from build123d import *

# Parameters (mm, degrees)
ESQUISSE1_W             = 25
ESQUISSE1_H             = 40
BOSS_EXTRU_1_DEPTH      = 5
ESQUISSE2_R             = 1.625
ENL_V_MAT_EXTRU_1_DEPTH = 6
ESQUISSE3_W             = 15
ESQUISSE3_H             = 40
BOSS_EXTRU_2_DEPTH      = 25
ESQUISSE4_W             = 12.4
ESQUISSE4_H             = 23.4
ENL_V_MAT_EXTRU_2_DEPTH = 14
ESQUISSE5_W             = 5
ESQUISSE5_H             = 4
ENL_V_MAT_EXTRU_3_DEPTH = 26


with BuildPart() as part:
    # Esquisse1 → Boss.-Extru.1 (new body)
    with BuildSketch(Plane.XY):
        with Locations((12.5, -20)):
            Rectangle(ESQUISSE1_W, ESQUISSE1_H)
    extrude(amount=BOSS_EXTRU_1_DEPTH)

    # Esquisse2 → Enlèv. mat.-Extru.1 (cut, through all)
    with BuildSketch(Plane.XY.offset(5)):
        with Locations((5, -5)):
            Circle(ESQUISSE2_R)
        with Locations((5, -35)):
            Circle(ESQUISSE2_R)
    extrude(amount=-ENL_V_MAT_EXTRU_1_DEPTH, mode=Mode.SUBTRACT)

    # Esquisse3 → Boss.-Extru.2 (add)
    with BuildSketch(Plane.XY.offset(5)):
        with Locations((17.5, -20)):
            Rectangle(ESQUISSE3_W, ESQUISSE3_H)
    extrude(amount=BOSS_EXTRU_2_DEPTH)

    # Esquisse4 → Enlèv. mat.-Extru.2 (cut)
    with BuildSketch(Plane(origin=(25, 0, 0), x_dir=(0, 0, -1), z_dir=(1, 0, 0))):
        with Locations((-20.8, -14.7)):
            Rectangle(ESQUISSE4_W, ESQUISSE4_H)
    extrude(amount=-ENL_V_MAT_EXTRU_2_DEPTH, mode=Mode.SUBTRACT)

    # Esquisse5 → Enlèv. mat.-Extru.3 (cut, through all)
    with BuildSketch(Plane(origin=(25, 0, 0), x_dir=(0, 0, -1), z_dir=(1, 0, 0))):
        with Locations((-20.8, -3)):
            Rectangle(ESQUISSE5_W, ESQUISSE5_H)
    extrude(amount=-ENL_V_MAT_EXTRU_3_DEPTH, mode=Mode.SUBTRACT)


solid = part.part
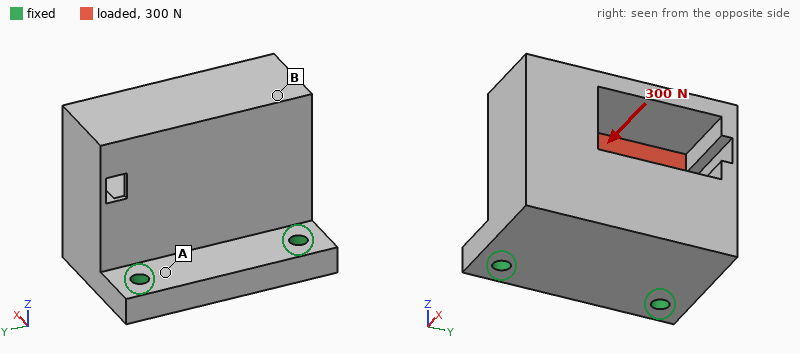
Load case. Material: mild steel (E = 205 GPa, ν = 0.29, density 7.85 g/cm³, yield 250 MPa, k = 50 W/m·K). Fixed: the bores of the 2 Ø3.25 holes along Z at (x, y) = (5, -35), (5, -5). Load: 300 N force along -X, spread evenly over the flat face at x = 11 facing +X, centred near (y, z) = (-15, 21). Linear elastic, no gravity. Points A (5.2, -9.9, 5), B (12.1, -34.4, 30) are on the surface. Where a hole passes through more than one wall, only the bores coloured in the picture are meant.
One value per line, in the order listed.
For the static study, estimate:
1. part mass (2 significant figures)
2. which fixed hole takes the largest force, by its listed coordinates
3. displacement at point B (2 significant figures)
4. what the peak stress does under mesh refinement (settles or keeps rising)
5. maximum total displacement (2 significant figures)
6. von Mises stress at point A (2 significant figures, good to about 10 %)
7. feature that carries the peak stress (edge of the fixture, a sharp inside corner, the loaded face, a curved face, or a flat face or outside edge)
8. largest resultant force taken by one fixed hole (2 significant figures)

120 g
(5, -5)
18 µm
keeps rising
22 µm
23 MPa
edge of the fixture
200 N
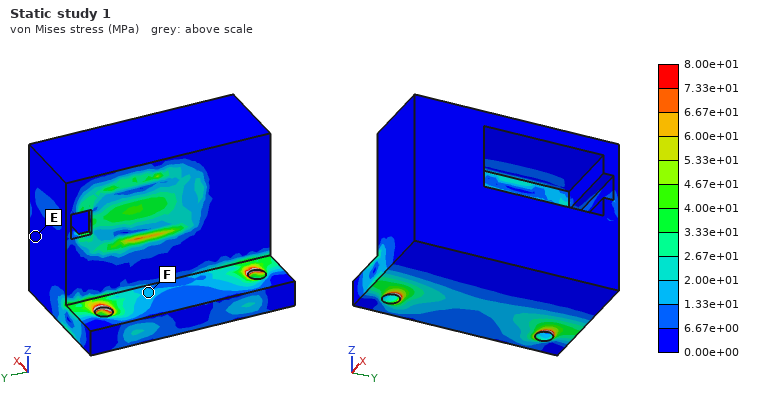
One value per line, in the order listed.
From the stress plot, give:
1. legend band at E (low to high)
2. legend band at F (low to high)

0.00e+00 to 6.67e+00 MPa
1.33e+01 to 2.00e+01 MPa
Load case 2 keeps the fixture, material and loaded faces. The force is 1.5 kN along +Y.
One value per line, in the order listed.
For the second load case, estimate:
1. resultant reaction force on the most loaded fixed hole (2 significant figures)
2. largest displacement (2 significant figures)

1.2 kN
12 µm
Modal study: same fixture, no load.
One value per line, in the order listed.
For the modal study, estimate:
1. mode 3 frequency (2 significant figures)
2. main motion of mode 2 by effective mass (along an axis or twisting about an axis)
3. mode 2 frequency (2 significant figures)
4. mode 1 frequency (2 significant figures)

12 kHz
along Y
8200 Hz
2600 Hz
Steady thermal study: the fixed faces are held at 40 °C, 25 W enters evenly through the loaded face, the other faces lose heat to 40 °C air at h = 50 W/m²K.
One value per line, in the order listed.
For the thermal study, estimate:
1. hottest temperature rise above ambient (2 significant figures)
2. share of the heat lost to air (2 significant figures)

82 K
34 %
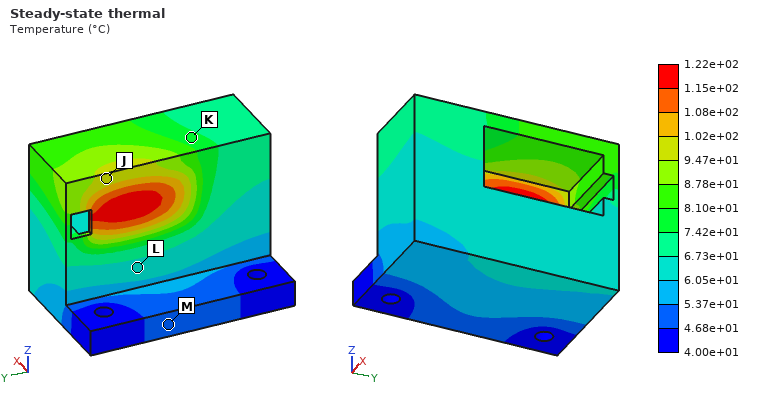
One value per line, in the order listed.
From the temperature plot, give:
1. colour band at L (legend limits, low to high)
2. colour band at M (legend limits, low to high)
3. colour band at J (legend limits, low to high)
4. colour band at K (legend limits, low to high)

6.05e+01 to 6.73e+01 °C
4.68e+01 to 5.37e+01 °C
9.47e+01 to 1.02e+02 °C
7.42e+01 to 8.10e+01 °C
